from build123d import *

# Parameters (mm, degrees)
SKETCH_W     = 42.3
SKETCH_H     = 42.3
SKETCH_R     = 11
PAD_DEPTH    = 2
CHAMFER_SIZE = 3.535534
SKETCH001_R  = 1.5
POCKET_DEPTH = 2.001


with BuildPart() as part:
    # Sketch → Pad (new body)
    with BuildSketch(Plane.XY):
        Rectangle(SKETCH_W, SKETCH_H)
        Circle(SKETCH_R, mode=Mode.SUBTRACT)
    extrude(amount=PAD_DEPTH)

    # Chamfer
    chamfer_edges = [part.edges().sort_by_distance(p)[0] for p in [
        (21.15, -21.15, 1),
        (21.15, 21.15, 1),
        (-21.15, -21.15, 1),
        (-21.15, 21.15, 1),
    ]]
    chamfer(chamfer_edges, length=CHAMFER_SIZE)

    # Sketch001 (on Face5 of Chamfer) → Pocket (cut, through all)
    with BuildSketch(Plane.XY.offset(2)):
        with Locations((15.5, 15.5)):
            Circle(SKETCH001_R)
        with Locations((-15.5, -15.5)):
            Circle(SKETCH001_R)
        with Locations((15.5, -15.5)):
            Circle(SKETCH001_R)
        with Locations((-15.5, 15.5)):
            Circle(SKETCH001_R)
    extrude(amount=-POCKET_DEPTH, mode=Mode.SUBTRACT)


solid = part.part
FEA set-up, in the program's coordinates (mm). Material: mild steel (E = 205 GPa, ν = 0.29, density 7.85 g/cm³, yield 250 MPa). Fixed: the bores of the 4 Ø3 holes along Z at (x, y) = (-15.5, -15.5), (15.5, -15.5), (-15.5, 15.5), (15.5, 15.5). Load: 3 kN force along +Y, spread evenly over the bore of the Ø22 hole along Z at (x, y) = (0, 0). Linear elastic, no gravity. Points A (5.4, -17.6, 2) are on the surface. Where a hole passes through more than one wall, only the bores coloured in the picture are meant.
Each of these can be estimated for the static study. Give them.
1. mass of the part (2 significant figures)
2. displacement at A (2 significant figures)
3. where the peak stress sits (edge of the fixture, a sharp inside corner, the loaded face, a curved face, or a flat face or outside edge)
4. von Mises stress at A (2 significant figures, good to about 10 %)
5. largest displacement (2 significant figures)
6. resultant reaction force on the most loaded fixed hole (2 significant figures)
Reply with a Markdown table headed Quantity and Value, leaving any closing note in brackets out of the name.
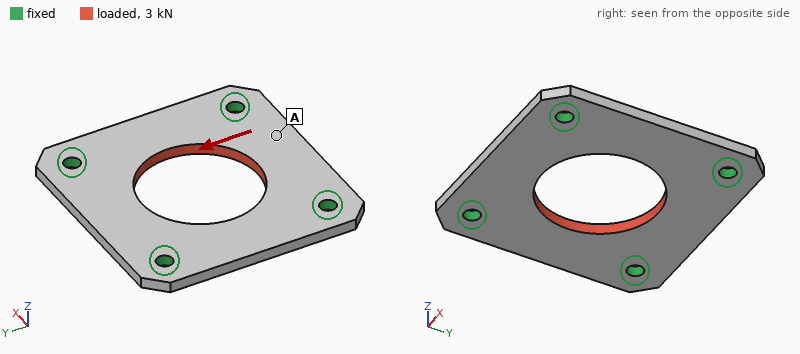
| Quantity | Value |
|---|---|
| mass of the part | 21 g |
| displacement at A | 3.4 µm |
| where the peak stress sits | edge of the fixture |
| von Mises stress at A | 22 MPa |
| largest displacement | 4.6 µm |
| resultant reaction force on the most loaded fixed hole | 770 N |
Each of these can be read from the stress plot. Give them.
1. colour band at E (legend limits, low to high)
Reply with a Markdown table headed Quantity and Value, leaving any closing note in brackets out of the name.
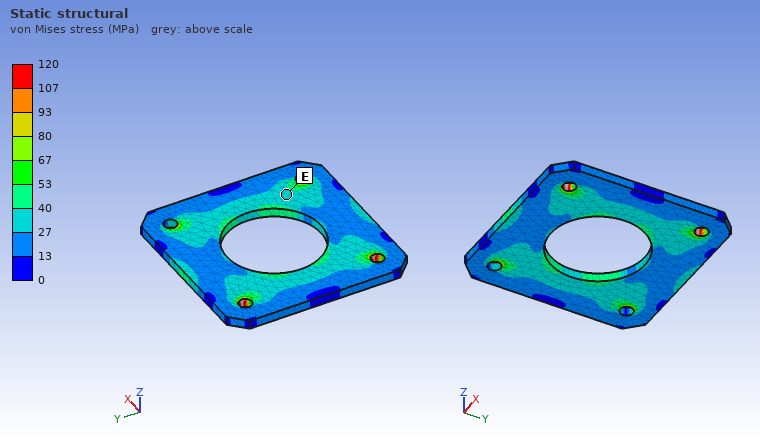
| Quantity | Value |
|---|---|
| colour band at E | 27 to 40 MPa |
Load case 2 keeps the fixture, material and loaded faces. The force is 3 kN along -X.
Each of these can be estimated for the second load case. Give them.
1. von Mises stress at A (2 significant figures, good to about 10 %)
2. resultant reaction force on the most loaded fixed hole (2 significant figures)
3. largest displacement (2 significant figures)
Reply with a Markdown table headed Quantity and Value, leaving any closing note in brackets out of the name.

| Quantity | Value |
|---|---|
| von Mises stress at A | 19 MPa |
| resultant reaction force on the most loaded fixed hole | 770 N |
| largest displacement | 4.6 µm |
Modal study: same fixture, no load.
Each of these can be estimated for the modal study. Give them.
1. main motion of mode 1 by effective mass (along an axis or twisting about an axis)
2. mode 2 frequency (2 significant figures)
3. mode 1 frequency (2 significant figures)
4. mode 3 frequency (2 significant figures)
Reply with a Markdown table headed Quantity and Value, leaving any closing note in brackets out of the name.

| Quantity | Value |
|---|---|
| main motion of mode 1 by effective mass | along Z |
| mode 2 frequency | 12 kHz |
| mode 1 frequency | 11 kHz |
| mode 3 frequency | 12 kHz |
